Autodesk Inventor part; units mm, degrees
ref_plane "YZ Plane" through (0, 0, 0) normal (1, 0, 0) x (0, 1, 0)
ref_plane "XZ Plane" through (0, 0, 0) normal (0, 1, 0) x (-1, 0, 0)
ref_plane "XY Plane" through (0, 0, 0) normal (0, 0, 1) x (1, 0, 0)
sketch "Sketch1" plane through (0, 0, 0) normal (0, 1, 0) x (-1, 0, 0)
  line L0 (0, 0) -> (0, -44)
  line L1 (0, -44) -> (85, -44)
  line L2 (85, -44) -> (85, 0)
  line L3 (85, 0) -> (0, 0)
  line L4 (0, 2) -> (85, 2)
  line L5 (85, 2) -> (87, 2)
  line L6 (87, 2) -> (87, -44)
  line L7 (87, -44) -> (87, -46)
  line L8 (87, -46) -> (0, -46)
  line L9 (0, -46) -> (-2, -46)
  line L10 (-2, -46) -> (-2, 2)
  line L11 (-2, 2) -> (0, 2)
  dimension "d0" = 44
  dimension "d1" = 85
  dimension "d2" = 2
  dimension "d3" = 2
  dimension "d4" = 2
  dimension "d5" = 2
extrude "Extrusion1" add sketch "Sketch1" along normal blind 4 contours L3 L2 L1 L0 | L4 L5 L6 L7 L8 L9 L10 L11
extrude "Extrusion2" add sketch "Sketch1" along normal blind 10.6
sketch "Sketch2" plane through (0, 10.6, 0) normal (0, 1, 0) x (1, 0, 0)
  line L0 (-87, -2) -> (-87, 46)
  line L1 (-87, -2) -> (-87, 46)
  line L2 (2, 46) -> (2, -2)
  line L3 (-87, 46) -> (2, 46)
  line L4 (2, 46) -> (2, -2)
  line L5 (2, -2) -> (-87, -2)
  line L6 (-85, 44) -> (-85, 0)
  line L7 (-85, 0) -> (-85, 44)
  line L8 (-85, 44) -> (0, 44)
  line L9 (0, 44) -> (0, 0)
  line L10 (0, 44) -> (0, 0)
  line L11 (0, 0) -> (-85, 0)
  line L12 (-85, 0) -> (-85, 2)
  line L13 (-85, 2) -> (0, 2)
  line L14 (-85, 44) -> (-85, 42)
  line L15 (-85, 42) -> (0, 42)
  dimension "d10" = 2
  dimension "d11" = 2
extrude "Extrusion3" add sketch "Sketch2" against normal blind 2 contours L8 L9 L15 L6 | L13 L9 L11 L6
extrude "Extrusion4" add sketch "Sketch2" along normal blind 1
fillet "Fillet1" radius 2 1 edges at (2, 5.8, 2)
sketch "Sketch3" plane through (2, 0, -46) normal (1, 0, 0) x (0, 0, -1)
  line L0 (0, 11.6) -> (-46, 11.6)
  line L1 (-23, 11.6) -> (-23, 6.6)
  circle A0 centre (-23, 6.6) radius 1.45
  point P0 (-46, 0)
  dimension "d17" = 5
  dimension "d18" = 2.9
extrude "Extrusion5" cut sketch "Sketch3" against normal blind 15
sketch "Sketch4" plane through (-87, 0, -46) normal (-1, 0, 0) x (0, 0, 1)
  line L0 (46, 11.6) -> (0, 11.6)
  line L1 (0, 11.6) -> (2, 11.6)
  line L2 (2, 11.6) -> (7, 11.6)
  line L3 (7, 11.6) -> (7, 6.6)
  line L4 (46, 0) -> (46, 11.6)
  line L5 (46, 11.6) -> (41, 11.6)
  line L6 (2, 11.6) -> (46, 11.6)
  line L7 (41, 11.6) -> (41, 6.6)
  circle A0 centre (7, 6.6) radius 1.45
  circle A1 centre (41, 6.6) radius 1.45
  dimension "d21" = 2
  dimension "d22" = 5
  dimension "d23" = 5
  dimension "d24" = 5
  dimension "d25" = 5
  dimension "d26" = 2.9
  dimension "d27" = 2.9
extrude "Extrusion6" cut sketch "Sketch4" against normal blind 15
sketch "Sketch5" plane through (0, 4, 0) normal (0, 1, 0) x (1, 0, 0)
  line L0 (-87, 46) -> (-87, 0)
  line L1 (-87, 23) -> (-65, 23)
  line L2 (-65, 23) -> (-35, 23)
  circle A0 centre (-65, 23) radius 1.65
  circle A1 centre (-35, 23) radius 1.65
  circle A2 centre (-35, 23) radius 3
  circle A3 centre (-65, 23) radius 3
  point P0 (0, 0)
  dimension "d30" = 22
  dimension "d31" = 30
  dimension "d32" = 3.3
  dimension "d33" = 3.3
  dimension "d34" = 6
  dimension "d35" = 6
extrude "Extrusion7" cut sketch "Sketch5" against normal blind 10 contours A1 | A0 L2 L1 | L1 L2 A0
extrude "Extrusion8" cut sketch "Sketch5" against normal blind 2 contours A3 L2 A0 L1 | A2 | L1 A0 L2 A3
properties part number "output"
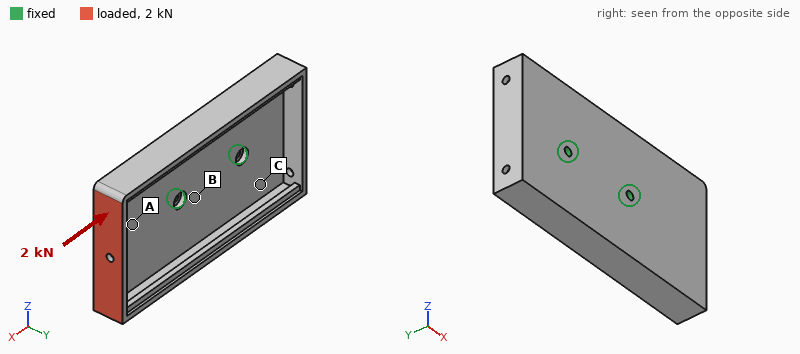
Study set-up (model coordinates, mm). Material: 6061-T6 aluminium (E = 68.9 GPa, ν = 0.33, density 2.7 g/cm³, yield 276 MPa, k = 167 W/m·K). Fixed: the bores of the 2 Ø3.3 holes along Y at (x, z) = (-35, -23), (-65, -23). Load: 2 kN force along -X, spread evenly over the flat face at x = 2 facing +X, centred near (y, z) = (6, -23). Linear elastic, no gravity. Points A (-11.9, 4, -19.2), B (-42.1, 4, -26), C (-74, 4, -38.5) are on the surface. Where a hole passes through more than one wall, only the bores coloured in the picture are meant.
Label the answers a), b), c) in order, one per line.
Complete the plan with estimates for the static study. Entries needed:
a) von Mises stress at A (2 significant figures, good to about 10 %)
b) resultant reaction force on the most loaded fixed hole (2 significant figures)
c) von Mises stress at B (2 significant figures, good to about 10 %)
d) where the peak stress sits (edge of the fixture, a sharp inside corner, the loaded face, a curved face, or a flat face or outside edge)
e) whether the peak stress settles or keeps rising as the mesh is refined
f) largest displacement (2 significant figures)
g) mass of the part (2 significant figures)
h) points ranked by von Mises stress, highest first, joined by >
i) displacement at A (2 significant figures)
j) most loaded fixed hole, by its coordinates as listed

a) 29 MPa
b) 1.2 kN
c) 16 MPa
d) edge of the fixture
e) keeps rising
f) 0.18 mm
g) 58 g
h) A > B > C
i) 0.062 mm
j) (-35, -23)
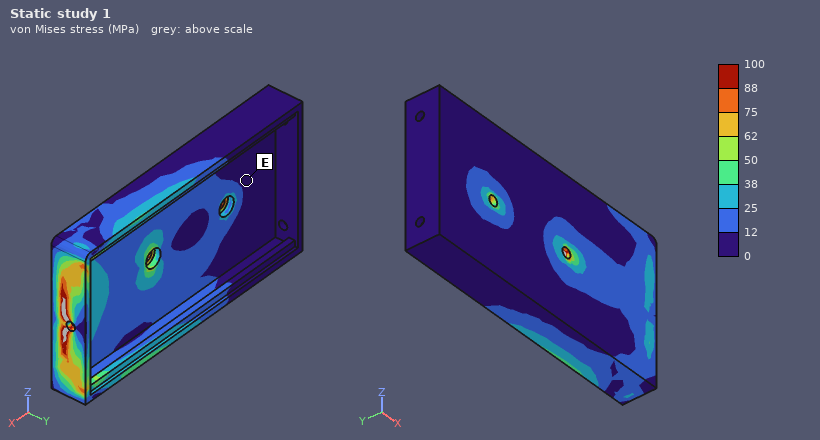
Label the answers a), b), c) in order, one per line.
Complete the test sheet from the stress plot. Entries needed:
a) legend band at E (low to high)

a) 0 to 12 MPa
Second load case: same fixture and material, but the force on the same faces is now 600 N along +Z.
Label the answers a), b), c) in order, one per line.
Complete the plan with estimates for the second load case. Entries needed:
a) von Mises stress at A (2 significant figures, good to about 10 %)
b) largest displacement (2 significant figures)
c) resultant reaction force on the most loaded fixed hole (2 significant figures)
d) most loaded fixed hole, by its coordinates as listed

a) 21 MPa
b) 0.15 mm
c) 1.3 kN
d) (-35, -23)
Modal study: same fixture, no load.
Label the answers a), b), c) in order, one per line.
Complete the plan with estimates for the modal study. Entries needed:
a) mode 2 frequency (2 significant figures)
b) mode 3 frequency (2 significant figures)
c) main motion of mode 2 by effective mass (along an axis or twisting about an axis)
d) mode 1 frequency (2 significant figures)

a) 2100 Hz
b) 2600 Hz
c) along Y
d) 1500 Hz
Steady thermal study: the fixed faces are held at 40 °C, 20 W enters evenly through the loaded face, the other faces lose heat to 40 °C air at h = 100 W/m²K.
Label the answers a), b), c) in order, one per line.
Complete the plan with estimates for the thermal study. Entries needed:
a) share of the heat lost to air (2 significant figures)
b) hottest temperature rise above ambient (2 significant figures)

a) 45 %
b) 24 K
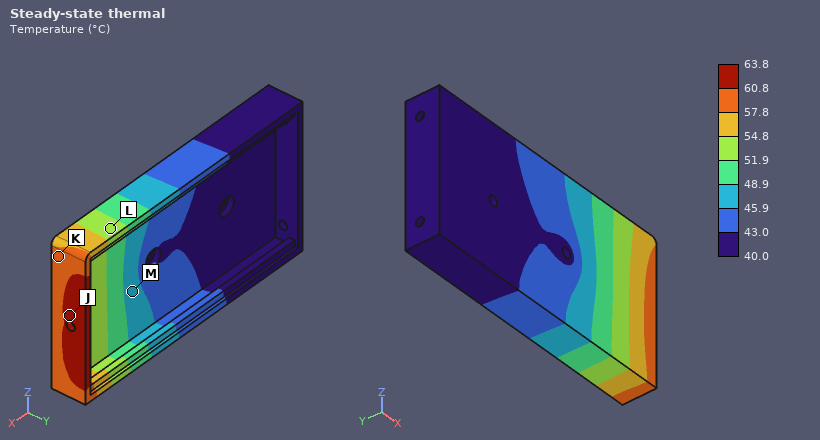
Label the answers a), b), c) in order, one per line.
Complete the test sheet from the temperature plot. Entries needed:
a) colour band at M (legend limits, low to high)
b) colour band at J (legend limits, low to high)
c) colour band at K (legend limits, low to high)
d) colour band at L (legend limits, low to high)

a) 45.9 to 48.9 °C
b) 60.8 to 63.8 °C
c) 57.8 to 60.8 °C
d) 51.9 to 54.8 °C
